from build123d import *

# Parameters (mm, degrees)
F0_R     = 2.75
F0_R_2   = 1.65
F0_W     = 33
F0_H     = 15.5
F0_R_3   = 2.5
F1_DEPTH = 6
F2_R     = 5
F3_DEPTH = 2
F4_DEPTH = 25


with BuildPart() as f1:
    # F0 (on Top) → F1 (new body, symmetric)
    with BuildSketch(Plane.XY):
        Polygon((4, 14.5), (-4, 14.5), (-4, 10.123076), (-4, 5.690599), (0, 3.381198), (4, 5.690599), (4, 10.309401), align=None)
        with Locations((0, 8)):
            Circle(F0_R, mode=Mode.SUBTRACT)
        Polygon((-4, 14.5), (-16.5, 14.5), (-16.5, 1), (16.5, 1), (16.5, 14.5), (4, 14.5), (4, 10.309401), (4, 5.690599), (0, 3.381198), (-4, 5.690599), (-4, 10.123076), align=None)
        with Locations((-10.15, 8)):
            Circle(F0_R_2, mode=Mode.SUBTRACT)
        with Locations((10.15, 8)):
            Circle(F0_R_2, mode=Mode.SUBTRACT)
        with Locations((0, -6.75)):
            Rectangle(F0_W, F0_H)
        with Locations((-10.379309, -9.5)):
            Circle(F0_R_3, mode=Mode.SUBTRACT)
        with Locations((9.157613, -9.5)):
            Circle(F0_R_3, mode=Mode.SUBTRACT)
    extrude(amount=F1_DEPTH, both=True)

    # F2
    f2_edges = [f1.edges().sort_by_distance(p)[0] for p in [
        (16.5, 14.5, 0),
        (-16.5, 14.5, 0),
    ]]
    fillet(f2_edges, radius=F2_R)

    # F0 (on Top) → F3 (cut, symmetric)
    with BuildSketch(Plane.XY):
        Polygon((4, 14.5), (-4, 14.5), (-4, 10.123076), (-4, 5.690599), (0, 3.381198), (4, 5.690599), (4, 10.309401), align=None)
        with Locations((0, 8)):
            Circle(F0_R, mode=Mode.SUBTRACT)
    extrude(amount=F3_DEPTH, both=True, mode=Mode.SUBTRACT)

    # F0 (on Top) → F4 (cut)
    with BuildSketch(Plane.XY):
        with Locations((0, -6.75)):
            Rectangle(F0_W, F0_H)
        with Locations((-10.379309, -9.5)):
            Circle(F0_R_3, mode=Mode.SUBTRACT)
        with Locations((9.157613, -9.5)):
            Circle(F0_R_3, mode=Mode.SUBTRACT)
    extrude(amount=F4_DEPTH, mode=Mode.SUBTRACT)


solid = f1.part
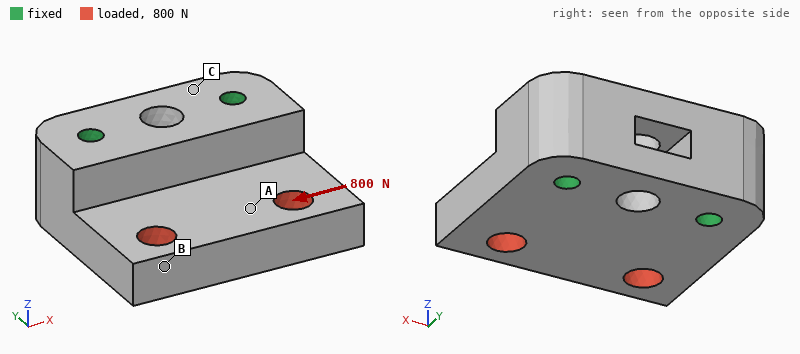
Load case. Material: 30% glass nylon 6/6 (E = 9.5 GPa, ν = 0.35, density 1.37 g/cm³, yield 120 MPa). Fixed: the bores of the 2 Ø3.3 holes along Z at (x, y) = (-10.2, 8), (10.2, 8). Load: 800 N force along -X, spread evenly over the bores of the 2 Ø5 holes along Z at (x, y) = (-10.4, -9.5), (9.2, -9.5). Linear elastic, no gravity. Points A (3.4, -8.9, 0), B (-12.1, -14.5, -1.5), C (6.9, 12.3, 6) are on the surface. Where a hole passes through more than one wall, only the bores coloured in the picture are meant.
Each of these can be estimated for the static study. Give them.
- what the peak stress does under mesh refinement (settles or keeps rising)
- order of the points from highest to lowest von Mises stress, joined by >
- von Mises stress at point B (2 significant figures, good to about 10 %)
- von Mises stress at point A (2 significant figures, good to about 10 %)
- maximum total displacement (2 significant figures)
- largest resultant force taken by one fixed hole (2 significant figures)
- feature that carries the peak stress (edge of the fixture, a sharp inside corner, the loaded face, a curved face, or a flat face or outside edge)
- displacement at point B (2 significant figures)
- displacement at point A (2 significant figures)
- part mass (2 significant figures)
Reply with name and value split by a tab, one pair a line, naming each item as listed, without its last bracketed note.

what the peak stress does under mesh refinement	keeps rising
order of the points from highest to lowest von Mises stress, joined by >	A > B > C
von Mises stress at point B	5.0 MPa
von Mises stress at point A	8.4 MPa
maximum total displacement	45 µm
largest resultant force taken by one fixed hole	710 N
feature that carries the peak stress	edge of the fixture
displacement at point B	42 µm
displacement at point A	29 µm
part mass	10 g
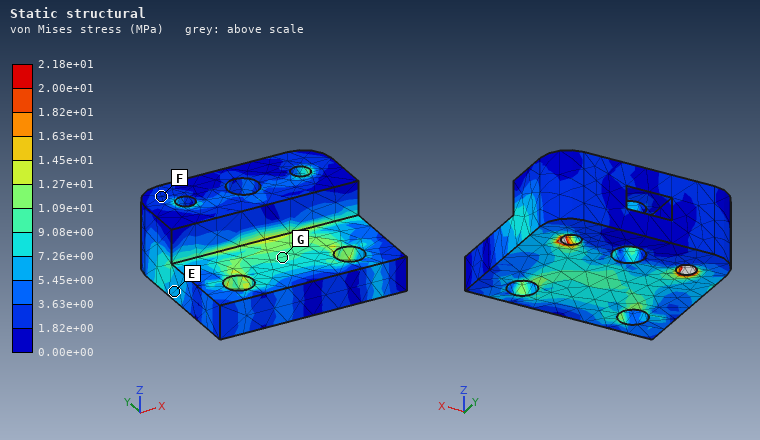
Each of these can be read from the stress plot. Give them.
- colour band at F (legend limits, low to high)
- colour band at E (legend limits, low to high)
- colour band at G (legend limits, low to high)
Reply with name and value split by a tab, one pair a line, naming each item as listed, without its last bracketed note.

colour band at F	1.82e+00 to 3.63e+00 MPa
colour band at E	5.45e+00 to 7.26e+00 MPa
colour band at G	9.08e+00 to 1.09e+01 MPa
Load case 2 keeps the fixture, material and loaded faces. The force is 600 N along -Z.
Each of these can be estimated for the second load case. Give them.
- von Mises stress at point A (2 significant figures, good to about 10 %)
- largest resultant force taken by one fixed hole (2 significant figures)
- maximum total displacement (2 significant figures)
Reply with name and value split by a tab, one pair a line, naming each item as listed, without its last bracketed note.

von Mises stress at point A	5.1 MPa
largest resultant force taken by one fixed hole	310 N
maximum total displacement	0.18 mm
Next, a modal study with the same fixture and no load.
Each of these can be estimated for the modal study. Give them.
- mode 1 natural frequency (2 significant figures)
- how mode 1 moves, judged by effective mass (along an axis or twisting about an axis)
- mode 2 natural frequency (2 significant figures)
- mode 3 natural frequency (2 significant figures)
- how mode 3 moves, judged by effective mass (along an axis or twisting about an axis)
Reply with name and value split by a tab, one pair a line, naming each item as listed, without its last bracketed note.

mode 1 natural frequency	6800 Hz
how mode 1 moves, judged by effective mass	along Z
mode 2 natural frequency	10 kHz
mode 3 natural frequency	14 kHz
how mode 3 moves, judged by effective mass	along X
